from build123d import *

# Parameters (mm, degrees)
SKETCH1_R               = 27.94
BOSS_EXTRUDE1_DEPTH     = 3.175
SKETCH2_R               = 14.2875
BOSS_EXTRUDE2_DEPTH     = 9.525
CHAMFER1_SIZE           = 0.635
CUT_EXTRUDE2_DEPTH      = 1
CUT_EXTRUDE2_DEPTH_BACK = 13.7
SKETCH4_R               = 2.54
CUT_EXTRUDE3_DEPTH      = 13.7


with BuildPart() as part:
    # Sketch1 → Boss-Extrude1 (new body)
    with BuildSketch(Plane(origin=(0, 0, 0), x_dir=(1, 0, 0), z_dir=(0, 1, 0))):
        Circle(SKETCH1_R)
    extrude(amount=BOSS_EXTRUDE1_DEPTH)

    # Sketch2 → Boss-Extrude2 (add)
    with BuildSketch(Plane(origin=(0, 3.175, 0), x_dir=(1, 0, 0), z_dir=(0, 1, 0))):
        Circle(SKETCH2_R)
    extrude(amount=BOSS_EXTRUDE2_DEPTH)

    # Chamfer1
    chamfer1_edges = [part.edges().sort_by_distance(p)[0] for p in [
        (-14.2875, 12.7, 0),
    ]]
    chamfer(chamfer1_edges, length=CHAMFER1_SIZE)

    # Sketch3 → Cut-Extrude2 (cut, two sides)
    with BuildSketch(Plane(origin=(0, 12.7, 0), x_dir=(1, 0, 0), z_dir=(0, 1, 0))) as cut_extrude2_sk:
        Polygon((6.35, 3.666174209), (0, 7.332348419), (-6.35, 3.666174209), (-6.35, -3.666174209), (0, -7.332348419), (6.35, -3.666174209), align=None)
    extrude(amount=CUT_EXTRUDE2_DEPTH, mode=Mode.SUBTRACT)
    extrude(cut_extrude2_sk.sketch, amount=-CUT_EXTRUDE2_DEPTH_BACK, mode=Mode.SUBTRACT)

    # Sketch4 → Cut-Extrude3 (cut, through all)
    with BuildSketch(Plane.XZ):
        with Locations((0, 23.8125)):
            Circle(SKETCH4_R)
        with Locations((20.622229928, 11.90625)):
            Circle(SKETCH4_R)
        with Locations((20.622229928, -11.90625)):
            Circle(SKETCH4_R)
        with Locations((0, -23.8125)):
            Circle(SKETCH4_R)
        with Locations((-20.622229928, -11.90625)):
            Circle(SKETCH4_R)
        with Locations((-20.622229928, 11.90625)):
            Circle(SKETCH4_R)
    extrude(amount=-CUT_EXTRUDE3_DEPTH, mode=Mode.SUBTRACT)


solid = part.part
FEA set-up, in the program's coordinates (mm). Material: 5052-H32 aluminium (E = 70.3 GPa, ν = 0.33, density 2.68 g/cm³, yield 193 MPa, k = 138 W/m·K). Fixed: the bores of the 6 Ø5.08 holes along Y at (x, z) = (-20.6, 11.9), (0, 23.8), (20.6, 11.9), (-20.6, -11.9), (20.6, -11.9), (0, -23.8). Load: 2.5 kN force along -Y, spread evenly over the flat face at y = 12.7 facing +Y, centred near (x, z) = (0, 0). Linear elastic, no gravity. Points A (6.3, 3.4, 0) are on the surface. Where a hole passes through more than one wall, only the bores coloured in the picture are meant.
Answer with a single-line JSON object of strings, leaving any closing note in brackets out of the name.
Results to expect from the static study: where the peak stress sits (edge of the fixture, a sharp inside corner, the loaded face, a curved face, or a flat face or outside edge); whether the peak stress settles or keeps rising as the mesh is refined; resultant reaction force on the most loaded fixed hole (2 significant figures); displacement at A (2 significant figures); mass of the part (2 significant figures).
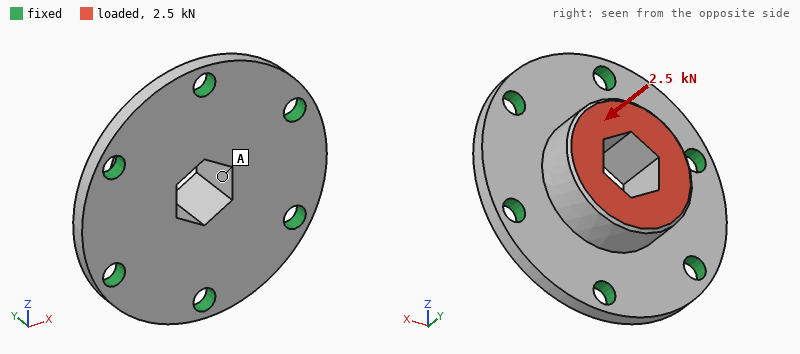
{"where the peak stress sits": "edge of the fixture", "whether the peak stress settles or keeps rising as the mesh is refined": "keeps rising", "resultant reaction force on the most loaded fixed hole": "480 N", "displacement at A": "17 µm", "mass of the part": "31 g"}
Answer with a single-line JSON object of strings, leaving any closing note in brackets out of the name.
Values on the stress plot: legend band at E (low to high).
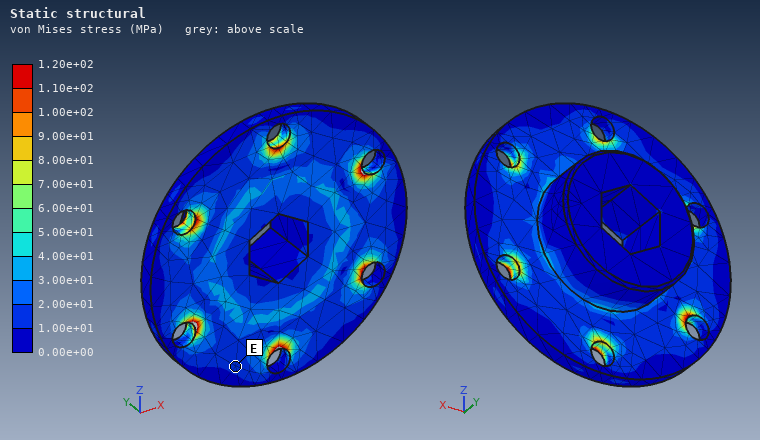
{"legend band at E": "1.00e+01 to 2.00e+01 MPa"}
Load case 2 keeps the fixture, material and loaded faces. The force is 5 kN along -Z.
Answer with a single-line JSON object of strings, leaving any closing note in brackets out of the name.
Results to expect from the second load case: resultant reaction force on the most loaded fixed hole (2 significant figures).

{"resultant reaction force on the most loaded fixed hole": "1.6 kN"}
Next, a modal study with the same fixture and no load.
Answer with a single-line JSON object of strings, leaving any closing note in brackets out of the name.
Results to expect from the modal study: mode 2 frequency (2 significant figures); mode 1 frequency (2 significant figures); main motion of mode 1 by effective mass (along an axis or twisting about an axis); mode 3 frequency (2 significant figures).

{"mode 2 frequency": "19 kHz", "mode 1 frequency": "14 kHz", "main motion of mode 1 by effective mass": "along Y", "mode 3 frequency": "19 kHz"}
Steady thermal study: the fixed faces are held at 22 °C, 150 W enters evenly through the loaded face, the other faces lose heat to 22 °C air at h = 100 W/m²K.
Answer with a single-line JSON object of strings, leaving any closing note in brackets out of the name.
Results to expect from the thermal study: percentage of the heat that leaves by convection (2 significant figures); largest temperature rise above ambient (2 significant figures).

{"percentage of the heat that leaves by convection": "8.4 %", "largest temperature rise above ambient": "58 K"}
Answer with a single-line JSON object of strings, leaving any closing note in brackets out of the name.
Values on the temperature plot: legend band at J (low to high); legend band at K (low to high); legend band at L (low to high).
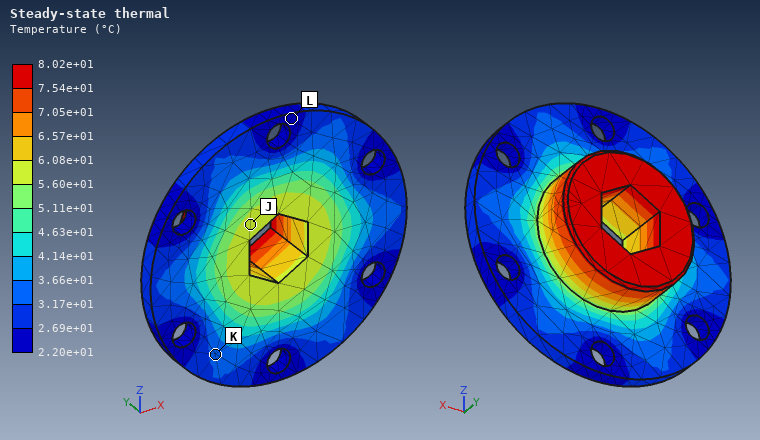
{"legend band at J": "5.60e+01 to 6.08e+01 °C", "legend band at K": "3.17e+01 to 3.66e+01 °C", "legend band at L": "2.20e+01 to 2.69e+01 °C"}
